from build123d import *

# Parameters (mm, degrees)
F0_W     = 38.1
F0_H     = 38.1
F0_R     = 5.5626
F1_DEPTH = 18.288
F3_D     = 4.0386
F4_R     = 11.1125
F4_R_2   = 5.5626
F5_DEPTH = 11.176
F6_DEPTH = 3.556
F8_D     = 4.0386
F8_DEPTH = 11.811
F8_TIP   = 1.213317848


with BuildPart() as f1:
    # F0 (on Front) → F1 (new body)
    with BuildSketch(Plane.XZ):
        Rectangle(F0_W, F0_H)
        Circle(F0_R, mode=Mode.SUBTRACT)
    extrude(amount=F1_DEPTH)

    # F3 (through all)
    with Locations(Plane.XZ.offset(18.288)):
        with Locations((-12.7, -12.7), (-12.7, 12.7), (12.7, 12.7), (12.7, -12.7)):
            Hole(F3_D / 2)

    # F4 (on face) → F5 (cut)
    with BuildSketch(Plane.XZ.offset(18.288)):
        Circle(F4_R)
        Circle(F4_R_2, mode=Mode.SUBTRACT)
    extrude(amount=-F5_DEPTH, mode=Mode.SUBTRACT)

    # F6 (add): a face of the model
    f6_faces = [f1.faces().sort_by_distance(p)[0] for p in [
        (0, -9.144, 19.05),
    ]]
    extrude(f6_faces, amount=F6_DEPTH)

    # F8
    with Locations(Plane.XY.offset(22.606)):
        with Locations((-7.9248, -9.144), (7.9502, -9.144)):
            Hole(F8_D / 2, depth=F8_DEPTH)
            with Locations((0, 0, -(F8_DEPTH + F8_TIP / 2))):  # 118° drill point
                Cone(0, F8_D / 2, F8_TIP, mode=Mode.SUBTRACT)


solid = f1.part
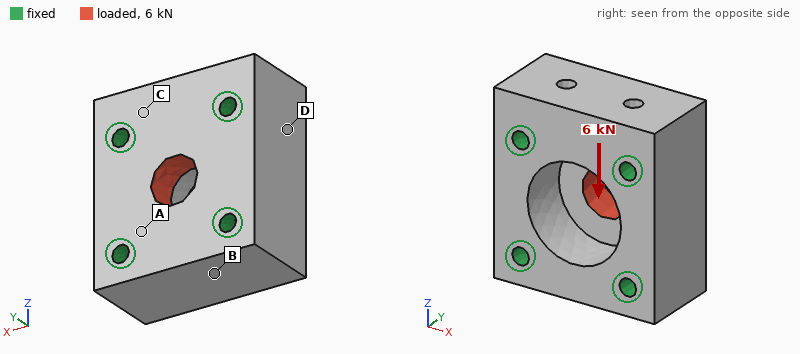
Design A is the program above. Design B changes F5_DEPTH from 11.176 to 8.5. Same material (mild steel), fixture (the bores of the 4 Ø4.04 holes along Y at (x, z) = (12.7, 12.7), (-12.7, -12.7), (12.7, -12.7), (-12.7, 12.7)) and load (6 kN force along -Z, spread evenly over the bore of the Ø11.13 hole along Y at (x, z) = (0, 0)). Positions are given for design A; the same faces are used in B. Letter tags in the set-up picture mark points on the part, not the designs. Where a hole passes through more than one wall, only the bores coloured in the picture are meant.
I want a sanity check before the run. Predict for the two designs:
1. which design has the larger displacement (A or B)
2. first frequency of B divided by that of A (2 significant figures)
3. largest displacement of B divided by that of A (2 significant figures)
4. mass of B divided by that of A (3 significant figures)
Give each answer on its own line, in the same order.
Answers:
A
1.0
0.76
1.03
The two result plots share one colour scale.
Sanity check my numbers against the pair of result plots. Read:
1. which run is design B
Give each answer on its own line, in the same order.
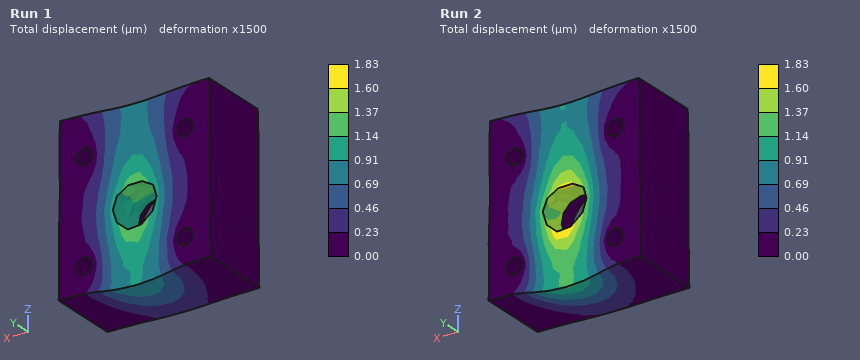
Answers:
Run 1
